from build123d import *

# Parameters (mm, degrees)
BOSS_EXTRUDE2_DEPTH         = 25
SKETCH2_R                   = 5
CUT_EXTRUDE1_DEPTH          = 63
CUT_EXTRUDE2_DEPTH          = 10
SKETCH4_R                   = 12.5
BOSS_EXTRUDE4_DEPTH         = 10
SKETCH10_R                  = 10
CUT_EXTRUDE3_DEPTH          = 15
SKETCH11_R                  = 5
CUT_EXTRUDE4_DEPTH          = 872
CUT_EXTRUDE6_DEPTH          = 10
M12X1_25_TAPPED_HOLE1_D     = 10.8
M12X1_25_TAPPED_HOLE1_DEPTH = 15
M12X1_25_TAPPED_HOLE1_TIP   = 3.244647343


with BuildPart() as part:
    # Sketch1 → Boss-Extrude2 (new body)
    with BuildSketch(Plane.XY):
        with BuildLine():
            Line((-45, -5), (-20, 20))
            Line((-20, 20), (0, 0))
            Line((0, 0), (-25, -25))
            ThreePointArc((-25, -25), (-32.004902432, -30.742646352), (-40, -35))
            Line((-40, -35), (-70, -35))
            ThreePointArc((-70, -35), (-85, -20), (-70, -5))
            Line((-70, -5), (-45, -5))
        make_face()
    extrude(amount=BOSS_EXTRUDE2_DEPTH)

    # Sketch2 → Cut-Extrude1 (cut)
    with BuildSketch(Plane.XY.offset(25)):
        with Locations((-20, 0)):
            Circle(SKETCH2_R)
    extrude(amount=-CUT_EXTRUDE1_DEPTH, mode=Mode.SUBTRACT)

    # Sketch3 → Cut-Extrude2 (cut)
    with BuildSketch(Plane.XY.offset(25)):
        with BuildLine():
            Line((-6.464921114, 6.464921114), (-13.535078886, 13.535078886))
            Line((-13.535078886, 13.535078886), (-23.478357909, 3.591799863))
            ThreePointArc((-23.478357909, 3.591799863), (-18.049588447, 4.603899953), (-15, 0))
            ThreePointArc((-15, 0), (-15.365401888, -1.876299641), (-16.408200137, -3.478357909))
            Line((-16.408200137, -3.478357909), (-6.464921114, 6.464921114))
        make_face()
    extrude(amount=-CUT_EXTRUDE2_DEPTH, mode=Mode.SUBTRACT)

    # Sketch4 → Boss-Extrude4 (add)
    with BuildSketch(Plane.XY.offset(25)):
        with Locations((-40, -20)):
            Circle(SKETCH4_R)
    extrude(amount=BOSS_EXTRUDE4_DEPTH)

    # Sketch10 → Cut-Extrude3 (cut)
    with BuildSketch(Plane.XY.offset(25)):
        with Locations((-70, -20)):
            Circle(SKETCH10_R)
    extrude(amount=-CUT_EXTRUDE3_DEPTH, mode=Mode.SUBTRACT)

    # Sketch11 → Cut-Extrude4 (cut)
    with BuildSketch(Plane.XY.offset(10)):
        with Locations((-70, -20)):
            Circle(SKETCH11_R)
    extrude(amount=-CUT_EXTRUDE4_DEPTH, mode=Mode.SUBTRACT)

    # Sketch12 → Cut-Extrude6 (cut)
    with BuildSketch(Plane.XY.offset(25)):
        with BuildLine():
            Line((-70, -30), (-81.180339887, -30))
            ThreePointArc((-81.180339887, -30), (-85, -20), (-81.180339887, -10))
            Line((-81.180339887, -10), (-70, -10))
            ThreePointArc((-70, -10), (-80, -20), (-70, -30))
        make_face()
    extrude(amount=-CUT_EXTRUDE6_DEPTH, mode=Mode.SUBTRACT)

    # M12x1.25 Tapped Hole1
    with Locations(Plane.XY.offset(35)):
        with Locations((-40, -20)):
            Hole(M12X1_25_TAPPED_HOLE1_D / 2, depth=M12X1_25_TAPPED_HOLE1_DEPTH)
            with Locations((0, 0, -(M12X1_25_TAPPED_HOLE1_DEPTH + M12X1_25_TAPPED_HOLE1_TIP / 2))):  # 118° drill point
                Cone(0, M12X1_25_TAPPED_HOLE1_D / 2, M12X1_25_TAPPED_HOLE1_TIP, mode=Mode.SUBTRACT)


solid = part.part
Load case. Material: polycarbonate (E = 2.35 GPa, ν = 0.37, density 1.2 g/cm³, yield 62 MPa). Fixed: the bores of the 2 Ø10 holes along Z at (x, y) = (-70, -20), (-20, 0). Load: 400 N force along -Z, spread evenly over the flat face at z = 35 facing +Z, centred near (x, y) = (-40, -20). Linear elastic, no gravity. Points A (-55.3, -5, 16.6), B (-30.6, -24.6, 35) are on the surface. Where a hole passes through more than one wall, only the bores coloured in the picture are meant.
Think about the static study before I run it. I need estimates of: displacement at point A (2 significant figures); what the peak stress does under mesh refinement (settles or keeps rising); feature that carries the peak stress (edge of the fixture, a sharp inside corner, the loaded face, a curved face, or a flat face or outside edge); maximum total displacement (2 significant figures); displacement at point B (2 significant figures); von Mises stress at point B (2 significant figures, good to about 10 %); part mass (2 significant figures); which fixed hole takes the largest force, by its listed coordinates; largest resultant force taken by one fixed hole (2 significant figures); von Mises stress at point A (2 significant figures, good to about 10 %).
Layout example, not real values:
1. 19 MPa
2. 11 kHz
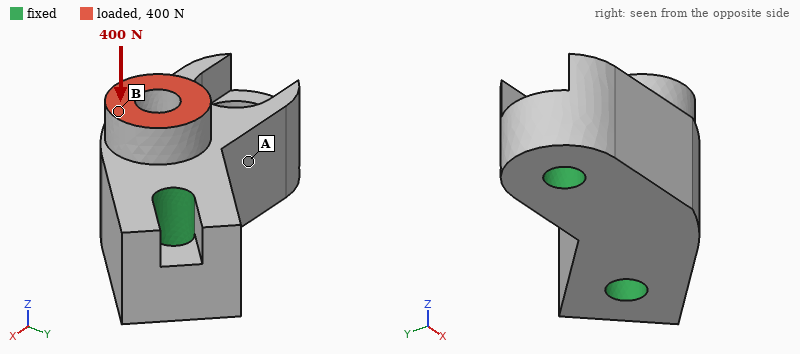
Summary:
1. 7.0 µm
2. keeps rising
3. edge of the fixture
4. 44 µm
5. 37 µm
6. 1.0 MPa
7. 66 g
8. (-20, 0)
9. 250 N
10. 0.42 MPa
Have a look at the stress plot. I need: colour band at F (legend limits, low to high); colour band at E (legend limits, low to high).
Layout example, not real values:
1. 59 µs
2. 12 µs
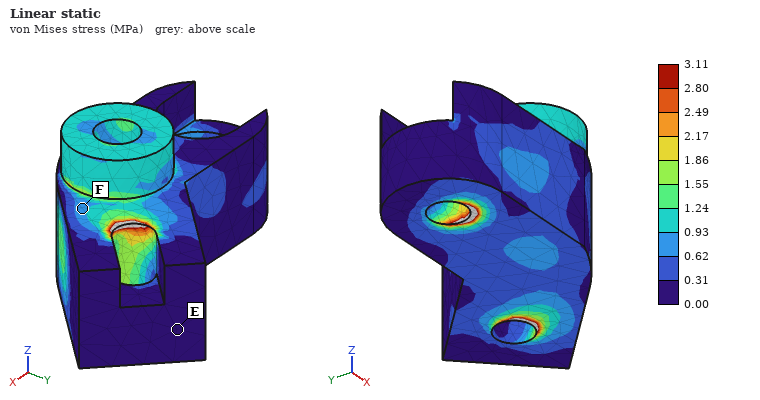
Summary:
1. 0.62 to 0.93 MPa
2. 0.00 to 0.31 MPa
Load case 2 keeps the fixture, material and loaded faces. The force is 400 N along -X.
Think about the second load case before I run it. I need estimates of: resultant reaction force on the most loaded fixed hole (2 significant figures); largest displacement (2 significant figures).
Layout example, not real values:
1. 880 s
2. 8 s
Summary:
1. 290 N
2. 72 µm
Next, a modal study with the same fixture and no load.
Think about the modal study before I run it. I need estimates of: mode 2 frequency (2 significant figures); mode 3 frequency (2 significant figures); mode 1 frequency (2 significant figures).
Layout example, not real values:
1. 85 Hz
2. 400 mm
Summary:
1. 5000 Hz
2. 6100 Hz
3. 3100 Hz
